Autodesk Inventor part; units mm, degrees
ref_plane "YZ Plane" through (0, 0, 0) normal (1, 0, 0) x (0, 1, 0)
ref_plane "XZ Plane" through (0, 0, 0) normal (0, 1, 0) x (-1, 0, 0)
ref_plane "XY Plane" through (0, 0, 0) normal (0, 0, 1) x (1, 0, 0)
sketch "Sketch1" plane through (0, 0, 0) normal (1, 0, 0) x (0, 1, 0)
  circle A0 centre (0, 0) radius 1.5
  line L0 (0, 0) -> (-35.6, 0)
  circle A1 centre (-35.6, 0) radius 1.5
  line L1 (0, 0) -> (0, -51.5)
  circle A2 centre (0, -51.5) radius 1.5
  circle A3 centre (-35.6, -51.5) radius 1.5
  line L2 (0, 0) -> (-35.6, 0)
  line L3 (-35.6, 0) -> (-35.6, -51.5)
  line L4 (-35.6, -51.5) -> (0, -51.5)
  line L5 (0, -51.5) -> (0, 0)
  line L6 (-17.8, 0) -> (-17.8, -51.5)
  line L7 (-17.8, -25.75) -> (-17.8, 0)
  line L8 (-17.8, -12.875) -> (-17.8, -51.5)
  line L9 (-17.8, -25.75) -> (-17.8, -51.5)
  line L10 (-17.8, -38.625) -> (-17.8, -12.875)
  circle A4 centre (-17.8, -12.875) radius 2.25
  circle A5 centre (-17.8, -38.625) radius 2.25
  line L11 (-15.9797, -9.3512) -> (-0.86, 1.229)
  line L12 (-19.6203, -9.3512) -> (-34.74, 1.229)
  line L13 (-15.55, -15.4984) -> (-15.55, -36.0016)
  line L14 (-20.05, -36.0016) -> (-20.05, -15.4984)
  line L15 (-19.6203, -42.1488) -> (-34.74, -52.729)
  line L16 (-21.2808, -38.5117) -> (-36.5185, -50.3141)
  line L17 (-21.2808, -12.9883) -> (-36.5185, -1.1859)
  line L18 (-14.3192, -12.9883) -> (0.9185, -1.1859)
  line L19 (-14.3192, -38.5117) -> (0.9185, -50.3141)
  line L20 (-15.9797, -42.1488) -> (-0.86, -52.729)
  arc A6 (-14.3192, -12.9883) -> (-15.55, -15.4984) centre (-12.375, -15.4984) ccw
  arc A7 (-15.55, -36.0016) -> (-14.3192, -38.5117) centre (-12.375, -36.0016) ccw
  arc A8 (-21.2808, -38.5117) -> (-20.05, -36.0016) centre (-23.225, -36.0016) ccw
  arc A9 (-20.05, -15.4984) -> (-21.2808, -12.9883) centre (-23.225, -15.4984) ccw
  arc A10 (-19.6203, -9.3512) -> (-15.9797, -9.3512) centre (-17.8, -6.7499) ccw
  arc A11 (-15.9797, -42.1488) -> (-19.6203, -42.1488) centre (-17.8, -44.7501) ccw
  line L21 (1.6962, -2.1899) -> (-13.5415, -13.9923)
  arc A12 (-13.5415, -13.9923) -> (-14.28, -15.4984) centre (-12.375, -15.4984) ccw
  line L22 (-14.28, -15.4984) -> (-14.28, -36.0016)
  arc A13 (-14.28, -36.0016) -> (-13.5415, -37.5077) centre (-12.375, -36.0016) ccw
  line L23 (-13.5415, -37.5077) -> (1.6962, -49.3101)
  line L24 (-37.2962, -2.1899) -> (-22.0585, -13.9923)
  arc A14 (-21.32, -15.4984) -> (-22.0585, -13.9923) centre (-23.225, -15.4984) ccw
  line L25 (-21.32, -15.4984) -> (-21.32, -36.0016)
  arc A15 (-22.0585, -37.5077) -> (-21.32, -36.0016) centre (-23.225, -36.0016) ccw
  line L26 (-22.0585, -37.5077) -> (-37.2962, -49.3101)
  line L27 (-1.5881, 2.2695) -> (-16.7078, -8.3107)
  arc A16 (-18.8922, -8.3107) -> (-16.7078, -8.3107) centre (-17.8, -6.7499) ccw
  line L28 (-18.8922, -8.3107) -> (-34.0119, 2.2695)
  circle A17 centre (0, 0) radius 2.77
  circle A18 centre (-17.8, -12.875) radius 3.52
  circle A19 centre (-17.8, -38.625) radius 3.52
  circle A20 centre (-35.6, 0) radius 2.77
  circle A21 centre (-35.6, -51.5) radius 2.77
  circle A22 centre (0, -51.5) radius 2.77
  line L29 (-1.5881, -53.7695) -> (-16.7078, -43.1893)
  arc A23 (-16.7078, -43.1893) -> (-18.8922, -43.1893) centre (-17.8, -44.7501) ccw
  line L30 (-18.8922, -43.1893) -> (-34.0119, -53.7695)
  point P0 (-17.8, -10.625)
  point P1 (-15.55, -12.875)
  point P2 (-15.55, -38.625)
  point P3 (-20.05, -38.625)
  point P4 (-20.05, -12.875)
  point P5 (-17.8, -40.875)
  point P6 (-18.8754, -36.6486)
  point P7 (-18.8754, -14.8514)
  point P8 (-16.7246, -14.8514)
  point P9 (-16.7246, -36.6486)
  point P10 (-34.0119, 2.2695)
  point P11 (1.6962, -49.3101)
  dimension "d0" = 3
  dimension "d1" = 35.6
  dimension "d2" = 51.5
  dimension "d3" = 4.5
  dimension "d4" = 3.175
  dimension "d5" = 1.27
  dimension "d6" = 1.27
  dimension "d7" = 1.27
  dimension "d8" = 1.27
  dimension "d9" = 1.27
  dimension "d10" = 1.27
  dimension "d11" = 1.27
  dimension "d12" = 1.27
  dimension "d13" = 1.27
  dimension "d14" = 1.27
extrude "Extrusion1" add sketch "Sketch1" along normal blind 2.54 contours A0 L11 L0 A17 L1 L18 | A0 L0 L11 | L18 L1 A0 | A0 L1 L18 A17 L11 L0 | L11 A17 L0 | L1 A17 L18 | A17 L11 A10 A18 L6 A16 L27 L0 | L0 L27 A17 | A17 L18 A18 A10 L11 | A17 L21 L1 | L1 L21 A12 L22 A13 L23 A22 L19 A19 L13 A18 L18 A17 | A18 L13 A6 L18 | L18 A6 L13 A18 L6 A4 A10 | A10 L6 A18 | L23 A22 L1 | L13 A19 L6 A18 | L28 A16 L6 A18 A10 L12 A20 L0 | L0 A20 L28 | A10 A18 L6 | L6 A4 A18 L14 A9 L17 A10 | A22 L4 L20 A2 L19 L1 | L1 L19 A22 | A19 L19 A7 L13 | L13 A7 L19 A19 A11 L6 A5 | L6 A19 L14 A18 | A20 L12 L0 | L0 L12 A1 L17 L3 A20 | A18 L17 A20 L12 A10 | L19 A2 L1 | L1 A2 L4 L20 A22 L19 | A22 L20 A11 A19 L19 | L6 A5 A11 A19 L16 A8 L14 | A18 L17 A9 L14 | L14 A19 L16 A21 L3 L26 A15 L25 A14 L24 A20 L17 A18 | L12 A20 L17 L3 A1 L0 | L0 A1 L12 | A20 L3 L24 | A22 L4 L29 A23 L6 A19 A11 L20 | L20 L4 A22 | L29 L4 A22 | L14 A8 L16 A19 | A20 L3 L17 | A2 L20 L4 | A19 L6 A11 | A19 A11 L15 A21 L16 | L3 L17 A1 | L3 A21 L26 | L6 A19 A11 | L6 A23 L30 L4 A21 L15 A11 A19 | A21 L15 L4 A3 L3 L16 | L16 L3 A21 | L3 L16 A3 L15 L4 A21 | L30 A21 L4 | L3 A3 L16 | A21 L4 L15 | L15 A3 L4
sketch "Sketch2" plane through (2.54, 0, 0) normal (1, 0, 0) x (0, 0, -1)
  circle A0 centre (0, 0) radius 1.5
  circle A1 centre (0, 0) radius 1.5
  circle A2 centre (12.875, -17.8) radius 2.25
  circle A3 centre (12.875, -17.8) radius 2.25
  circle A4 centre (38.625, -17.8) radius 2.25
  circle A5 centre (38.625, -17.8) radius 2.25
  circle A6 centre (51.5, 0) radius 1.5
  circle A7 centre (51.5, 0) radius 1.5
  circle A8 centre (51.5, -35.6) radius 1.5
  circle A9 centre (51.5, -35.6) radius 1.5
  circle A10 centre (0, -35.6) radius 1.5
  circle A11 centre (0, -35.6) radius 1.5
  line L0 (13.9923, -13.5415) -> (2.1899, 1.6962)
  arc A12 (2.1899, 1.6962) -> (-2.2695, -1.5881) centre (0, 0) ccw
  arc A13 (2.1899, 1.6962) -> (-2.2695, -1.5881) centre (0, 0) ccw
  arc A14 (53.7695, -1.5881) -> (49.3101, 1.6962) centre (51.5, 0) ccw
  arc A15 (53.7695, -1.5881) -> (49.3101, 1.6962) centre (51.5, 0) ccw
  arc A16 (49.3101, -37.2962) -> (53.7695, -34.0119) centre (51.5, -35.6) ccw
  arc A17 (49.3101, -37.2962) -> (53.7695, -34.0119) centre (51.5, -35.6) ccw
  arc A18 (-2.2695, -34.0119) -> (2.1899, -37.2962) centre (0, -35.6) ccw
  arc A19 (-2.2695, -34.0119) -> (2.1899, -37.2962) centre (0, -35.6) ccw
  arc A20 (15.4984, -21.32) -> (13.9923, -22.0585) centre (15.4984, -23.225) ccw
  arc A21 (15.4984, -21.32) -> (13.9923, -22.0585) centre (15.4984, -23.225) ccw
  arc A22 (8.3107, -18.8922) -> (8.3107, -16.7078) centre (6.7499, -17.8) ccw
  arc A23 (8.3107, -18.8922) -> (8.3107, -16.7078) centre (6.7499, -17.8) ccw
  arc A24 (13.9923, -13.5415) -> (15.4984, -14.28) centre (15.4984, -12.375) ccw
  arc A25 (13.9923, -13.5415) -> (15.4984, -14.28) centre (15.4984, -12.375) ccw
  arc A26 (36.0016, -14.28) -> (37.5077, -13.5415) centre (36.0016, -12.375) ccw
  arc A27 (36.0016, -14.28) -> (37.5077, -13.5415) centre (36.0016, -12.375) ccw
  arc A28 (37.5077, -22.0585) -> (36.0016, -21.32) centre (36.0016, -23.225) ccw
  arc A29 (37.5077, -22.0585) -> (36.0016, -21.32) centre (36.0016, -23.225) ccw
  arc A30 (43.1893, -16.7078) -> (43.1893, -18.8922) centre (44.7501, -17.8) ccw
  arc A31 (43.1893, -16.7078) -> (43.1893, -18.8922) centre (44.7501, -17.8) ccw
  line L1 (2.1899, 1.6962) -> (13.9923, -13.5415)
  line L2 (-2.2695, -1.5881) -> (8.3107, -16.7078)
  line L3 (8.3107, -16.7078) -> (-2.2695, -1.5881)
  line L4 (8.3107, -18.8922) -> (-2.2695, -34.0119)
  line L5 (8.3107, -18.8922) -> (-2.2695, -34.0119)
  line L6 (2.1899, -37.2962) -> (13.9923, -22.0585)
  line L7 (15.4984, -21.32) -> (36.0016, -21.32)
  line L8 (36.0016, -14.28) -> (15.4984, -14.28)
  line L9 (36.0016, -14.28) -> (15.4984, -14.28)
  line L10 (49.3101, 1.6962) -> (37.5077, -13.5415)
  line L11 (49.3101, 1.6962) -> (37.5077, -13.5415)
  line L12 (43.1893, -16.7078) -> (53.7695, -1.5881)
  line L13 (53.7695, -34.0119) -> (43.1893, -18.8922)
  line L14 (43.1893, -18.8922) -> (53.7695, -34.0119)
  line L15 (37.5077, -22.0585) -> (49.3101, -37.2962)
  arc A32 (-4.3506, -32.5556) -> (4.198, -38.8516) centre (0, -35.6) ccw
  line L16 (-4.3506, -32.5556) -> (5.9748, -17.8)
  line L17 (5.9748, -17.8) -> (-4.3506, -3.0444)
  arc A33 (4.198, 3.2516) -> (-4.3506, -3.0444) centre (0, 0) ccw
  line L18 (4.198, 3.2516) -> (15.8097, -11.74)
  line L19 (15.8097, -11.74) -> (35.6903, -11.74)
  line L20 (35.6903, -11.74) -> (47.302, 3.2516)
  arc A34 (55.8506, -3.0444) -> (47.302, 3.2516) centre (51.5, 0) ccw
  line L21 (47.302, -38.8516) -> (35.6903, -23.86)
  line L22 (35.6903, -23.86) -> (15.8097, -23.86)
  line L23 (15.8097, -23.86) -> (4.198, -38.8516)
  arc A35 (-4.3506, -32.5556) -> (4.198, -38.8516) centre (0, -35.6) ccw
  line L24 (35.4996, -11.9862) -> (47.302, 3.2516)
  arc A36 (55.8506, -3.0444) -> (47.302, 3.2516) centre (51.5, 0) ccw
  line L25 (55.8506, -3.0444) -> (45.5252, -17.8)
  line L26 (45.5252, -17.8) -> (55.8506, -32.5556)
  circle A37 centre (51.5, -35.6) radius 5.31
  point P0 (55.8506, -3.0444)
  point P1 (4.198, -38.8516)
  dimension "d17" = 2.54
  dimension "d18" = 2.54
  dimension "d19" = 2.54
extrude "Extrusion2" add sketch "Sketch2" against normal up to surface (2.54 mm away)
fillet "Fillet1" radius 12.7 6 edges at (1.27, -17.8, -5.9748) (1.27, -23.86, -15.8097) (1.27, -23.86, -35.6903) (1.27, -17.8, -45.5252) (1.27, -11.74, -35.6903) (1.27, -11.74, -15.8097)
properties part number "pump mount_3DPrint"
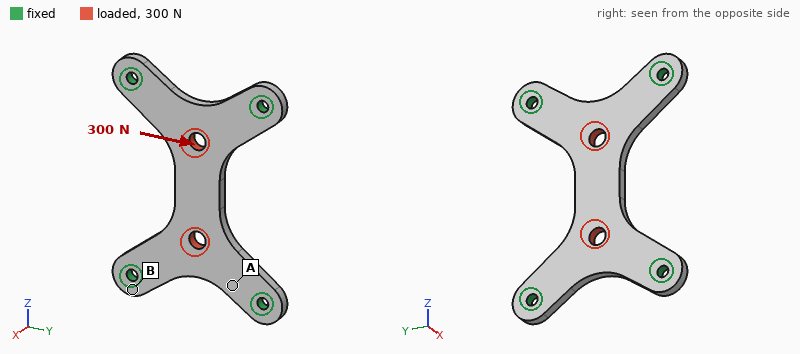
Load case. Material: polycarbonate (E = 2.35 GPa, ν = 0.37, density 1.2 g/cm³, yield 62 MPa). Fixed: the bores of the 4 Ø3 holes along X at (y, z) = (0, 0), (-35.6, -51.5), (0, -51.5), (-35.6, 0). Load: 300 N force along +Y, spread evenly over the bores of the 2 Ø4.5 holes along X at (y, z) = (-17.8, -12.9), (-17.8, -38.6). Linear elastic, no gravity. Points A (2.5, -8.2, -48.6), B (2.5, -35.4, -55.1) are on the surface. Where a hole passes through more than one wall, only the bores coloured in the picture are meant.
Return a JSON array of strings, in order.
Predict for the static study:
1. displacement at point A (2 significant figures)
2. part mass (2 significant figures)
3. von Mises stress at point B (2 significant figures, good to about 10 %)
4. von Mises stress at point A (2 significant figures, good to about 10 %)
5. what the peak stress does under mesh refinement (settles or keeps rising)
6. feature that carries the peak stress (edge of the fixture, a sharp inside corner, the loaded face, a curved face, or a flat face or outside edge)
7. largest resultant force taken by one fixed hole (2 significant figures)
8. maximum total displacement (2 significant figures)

["13 µm", "4.1 g", "1.3 MPa", "3.0 MPa", "keeps rising", "edge of the fixture", "92 N", "53 µm"]
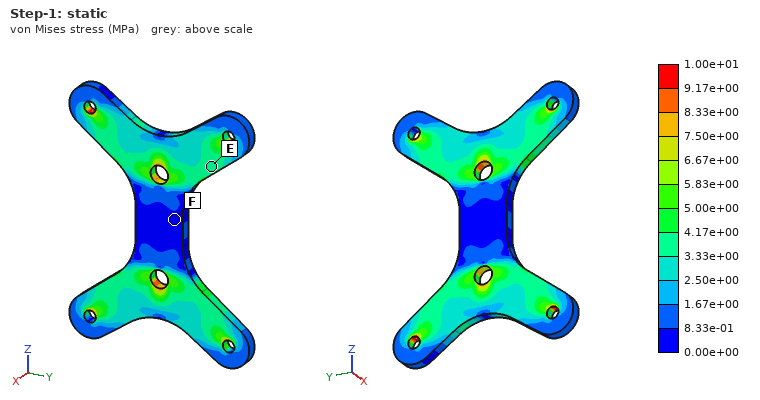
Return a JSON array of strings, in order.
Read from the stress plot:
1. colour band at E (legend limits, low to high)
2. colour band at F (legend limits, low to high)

["3.33e+00 to 4.17e+00 MPa", "0.00e+00 to 8.33e-01 MPa"]
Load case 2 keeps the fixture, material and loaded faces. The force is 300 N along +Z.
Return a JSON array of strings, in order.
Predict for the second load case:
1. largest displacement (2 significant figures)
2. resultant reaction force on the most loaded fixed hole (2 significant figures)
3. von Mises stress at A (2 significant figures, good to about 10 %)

["66 µm", "100 N", "3.7 MPa"]
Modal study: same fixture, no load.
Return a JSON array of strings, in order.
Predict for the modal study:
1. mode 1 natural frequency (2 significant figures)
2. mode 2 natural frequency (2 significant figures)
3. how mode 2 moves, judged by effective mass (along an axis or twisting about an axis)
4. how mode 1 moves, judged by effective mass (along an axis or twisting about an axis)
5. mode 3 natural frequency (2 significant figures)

["1200 Hz", "2500 Hz", "twisting about Y", "along X", "3900 Hz"]
